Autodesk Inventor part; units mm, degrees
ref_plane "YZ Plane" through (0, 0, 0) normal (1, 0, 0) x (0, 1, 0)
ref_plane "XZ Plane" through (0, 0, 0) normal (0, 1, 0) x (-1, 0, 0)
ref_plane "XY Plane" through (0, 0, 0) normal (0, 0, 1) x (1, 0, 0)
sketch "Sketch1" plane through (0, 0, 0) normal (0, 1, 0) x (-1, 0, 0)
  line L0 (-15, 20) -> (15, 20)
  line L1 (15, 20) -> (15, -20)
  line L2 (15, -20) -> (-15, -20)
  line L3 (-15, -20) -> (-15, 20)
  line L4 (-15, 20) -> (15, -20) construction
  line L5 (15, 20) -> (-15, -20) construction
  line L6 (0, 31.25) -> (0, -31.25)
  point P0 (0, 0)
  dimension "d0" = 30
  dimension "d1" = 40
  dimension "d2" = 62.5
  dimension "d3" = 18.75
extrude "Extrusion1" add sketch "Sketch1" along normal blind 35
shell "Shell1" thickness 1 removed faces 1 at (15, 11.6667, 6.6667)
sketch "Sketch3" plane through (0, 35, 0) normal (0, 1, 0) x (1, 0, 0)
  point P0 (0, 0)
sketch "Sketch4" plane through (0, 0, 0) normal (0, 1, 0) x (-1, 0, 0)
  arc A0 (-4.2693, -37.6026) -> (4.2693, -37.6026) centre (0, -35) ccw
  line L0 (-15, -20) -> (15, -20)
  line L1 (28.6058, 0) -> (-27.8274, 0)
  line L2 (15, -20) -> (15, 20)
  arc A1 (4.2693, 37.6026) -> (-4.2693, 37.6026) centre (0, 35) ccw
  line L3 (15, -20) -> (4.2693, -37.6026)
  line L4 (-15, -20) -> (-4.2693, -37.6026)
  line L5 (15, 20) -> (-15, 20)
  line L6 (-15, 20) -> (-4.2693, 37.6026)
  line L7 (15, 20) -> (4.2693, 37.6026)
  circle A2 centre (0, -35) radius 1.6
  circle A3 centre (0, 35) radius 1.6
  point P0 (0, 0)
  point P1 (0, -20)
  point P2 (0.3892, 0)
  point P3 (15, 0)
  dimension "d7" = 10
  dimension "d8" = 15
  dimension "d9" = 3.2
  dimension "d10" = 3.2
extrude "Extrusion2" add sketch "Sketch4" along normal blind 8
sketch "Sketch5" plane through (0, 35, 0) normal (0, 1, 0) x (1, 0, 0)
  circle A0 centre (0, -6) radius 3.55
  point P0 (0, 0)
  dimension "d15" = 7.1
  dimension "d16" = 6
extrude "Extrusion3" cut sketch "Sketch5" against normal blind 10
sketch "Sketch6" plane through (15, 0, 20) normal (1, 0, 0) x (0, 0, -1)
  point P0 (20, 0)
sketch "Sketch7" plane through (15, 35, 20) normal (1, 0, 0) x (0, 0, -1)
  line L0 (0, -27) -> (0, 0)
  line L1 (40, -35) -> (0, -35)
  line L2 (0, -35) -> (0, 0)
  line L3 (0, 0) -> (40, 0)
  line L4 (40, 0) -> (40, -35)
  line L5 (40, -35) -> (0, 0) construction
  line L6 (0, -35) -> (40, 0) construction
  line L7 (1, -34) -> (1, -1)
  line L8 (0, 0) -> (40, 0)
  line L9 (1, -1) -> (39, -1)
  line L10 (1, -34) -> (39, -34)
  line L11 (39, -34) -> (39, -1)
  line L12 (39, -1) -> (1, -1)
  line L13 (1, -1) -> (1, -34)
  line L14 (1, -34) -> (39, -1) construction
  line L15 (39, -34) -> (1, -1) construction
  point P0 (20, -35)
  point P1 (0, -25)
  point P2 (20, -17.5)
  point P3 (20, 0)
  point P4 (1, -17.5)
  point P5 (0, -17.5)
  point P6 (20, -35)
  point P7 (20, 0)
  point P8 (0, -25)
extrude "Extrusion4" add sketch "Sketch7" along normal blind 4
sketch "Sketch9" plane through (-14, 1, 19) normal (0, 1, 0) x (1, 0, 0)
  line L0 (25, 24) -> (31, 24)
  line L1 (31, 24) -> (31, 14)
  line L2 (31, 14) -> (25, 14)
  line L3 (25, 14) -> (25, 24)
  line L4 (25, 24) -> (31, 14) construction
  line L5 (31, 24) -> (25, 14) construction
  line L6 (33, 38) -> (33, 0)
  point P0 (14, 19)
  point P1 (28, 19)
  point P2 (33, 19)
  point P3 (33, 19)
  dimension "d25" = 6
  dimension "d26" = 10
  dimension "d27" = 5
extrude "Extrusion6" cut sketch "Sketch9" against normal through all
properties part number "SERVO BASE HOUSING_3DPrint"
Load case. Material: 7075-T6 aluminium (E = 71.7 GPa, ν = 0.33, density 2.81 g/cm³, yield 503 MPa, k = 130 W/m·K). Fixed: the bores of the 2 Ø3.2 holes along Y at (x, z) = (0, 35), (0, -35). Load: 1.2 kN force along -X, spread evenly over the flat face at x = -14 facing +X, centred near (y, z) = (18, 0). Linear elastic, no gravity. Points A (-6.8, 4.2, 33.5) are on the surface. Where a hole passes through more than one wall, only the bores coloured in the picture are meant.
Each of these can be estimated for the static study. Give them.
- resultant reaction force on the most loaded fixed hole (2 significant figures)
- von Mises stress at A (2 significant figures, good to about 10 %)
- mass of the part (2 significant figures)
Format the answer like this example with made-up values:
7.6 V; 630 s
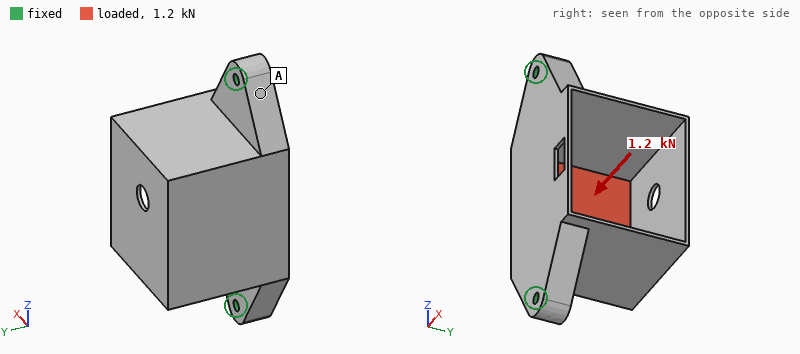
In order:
650 N; 32 MPa; 33 g
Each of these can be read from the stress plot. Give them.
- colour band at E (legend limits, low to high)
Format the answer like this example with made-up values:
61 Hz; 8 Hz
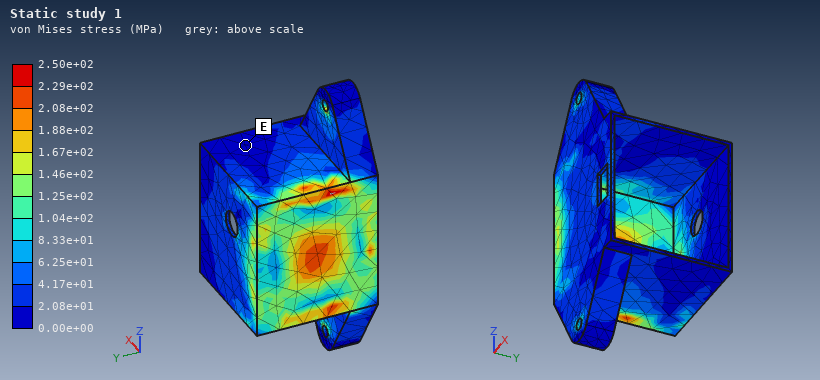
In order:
0.00e+00 to 2.08e+01 MPa
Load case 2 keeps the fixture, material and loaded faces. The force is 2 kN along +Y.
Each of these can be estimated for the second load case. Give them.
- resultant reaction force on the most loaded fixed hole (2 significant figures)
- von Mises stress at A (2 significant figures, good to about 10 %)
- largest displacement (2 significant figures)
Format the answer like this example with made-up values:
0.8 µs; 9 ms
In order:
1.0 kN; 52 MPa; 0.17 mm
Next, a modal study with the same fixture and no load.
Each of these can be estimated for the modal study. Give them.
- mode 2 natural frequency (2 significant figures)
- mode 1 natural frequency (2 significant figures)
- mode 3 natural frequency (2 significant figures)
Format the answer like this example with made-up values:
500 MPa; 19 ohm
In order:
3000 Hz; 2900 Hz; 3900 Hz
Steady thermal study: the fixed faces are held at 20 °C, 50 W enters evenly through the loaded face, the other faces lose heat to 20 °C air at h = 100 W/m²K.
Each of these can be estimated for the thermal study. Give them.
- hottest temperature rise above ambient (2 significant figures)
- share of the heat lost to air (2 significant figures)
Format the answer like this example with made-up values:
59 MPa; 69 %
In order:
65 K; 55 %
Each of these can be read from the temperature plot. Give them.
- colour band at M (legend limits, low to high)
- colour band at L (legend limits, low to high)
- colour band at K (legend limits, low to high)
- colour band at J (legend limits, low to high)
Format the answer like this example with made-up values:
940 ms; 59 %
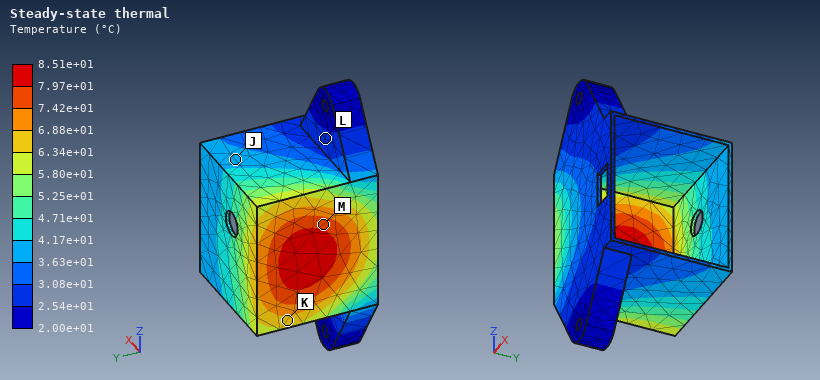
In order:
7.42e+01 to 7.97e+01 °C; 2.54e+01 to 3.08e+01 °C; 6.34e+01 to 6.88e+01 °C; 3.63e+01 to 4.17e+01 °C
